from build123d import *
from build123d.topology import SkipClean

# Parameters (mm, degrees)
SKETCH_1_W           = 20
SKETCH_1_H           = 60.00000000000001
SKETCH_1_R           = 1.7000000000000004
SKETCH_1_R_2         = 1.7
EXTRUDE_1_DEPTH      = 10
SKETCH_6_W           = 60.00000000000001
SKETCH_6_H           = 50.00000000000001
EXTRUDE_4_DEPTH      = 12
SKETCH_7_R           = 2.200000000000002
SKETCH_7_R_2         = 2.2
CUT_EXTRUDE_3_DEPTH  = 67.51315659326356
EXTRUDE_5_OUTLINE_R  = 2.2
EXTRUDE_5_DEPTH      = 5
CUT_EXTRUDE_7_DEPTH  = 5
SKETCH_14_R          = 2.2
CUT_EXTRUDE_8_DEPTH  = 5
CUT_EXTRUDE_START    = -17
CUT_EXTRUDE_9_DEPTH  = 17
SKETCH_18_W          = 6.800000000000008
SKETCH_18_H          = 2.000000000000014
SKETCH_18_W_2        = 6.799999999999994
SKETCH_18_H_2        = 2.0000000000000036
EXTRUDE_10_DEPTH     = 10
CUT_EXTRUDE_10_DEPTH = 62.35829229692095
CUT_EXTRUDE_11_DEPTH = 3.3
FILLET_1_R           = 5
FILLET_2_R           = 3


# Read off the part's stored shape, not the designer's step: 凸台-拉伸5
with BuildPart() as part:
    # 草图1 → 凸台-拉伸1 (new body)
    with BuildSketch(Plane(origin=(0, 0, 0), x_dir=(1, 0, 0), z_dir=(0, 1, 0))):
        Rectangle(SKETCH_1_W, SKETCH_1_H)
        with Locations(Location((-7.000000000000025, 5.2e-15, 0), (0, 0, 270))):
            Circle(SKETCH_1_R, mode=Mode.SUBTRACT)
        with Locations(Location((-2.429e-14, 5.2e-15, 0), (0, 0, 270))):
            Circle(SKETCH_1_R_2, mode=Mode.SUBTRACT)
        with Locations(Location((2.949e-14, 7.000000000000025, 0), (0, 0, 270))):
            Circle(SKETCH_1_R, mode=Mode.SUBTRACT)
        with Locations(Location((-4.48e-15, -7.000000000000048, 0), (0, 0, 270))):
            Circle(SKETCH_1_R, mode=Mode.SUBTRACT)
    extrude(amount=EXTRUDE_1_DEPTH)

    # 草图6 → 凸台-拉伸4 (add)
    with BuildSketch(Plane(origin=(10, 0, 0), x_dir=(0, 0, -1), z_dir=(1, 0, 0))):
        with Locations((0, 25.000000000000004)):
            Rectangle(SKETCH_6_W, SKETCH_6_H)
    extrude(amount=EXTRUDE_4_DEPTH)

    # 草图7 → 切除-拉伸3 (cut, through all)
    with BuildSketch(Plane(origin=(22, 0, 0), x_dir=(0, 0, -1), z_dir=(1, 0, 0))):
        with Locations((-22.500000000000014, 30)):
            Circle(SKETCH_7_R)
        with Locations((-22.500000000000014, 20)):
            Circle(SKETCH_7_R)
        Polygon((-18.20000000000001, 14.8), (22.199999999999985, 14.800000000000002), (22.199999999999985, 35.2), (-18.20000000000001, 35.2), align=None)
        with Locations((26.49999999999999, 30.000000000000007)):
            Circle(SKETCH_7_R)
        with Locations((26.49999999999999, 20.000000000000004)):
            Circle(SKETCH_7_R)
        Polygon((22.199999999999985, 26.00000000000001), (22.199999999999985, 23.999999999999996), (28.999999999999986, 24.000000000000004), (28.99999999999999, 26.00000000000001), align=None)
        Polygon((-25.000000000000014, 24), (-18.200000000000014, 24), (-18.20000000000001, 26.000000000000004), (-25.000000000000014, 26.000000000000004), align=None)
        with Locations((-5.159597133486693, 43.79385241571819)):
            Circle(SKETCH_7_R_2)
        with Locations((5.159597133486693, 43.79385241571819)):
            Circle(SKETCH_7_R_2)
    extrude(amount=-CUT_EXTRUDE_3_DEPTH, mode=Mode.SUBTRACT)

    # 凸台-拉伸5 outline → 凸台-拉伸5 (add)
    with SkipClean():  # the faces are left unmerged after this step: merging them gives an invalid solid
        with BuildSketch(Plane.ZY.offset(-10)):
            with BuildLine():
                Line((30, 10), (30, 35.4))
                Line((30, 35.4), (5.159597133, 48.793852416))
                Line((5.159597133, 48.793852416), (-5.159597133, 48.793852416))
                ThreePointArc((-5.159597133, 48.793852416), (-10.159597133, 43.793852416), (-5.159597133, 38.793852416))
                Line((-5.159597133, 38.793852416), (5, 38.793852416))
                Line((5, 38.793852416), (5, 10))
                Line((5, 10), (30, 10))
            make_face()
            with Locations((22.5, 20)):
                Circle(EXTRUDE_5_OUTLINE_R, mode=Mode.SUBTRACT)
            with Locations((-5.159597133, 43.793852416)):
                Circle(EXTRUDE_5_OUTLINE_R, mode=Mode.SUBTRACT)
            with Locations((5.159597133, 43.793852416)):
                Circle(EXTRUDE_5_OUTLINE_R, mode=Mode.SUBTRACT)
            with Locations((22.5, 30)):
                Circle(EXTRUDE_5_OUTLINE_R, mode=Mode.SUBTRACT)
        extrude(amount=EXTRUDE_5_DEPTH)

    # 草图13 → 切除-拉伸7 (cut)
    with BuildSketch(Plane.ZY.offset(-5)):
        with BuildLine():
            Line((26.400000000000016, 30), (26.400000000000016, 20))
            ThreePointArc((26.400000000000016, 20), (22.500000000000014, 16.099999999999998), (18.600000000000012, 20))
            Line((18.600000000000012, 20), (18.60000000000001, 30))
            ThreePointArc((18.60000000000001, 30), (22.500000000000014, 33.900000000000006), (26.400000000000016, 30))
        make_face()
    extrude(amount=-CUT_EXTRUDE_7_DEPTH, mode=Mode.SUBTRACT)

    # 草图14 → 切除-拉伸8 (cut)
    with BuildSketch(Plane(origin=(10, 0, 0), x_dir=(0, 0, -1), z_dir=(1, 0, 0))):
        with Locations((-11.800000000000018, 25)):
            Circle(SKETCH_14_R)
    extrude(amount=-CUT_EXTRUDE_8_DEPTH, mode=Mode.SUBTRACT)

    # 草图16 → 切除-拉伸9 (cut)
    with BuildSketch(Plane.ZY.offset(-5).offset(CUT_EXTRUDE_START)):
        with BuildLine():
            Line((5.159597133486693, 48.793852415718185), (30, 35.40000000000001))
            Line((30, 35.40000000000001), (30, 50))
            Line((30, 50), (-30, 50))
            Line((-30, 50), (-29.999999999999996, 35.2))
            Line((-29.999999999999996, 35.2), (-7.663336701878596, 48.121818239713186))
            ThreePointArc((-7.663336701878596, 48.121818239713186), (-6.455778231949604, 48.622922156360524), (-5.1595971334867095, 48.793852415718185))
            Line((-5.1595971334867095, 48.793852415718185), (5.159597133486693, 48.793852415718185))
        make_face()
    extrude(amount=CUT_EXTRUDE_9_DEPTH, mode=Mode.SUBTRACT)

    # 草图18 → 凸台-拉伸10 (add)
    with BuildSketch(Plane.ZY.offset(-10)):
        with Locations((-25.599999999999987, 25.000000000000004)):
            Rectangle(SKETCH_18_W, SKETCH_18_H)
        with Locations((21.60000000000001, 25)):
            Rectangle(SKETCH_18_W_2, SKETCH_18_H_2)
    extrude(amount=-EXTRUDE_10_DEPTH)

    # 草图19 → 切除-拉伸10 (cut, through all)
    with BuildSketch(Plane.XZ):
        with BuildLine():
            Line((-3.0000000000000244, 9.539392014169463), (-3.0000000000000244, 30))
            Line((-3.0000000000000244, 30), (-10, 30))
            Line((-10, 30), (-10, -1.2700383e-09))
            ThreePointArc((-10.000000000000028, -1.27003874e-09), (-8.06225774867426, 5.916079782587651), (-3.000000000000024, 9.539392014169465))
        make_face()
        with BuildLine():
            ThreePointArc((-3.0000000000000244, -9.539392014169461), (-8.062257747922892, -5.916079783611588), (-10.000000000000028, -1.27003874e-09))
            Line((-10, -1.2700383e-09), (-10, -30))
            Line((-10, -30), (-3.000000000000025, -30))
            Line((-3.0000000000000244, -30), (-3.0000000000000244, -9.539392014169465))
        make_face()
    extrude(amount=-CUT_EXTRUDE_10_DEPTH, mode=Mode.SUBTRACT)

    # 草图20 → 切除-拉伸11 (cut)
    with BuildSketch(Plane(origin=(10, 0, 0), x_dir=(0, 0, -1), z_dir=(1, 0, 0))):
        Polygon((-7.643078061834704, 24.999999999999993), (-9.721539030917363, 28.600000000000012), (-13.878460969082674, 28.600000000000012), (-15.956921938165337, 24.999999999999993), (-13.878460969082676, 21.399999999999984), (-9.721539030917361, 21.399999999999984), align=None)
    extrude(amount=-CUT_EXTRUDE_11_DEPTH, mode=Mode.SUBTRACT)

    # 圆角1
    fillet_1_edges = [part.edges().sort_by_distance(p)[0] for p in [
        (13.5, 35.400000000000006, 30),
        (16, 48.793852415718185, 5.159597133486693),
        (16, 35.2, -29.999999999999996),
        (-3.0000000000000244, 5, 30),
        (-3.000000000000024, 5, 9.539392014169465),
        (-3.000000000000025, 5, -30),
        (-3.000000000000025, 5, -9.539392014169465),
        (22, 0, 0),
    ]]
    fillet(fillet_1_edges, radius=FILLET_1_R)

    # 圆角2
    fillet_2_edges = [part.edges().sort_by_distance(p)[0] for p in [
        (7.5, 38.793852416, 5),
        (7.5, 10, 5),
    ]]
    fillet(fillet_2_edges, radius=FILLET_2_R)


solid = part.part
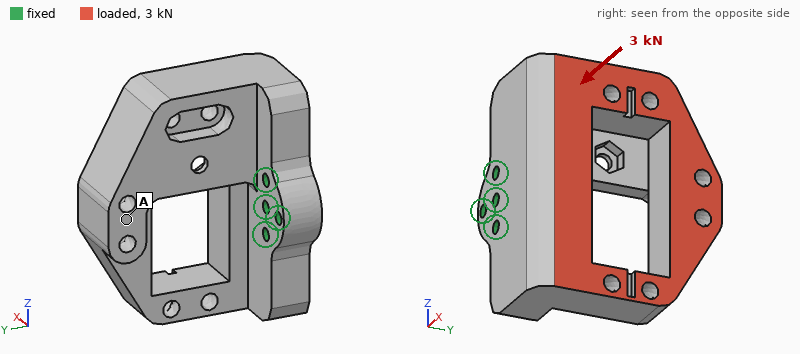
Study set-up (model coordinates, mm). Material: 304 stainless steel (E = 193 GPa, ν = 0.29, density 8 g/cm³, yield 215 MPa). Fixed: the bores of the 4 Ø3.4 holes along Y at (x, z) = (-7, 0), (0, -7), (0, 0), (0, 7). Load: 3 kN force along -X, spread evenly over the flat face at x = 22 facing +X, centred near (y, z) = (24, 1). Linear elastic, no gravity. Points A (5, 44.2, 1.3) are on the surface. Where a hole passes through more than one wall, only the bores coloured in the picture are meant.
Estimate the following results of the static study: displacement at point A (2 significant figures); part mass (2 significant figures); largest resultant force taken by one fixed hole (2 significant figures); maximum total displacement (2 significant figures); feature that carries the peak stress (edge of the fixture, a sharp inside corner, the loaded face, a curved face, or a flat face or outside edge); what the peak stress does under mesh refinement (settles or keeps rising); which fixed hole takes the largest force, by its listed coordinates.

74 µm
260 g
1.6 kN
90 µm
edge of the fixture
keeps rising
(0, 7)
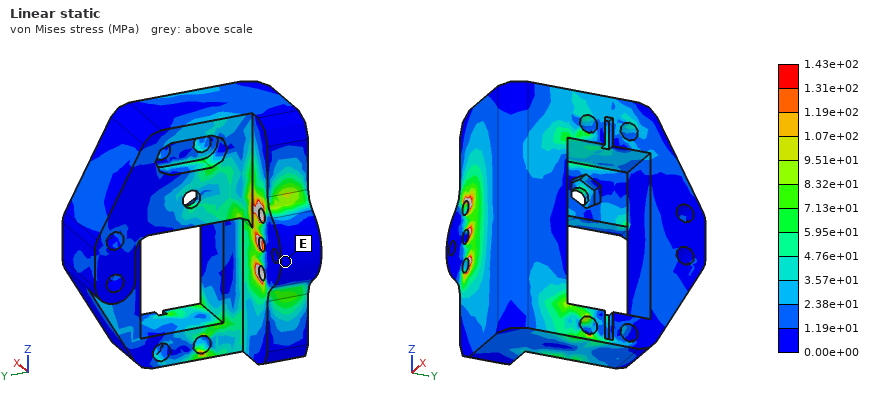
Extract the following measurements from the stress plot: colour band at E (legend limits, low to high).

0.00e+00 to 1.19e+01 MPa
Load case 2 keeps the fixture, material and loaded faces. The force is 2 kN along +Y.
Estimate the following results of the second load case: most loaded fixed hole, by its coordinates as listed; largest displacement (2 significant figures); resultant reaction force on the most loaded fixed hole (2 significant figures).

(0, 7)
50 µm
820 N
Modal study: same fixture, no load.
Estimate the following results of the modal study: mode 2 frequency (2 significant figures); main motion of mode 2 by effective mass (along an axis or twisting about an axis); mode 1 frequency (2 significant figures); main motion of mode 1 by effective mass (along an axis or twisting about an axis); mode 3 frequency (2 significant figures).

3500 Hz
along Z
2600 Hz
along X
5800 Hz
